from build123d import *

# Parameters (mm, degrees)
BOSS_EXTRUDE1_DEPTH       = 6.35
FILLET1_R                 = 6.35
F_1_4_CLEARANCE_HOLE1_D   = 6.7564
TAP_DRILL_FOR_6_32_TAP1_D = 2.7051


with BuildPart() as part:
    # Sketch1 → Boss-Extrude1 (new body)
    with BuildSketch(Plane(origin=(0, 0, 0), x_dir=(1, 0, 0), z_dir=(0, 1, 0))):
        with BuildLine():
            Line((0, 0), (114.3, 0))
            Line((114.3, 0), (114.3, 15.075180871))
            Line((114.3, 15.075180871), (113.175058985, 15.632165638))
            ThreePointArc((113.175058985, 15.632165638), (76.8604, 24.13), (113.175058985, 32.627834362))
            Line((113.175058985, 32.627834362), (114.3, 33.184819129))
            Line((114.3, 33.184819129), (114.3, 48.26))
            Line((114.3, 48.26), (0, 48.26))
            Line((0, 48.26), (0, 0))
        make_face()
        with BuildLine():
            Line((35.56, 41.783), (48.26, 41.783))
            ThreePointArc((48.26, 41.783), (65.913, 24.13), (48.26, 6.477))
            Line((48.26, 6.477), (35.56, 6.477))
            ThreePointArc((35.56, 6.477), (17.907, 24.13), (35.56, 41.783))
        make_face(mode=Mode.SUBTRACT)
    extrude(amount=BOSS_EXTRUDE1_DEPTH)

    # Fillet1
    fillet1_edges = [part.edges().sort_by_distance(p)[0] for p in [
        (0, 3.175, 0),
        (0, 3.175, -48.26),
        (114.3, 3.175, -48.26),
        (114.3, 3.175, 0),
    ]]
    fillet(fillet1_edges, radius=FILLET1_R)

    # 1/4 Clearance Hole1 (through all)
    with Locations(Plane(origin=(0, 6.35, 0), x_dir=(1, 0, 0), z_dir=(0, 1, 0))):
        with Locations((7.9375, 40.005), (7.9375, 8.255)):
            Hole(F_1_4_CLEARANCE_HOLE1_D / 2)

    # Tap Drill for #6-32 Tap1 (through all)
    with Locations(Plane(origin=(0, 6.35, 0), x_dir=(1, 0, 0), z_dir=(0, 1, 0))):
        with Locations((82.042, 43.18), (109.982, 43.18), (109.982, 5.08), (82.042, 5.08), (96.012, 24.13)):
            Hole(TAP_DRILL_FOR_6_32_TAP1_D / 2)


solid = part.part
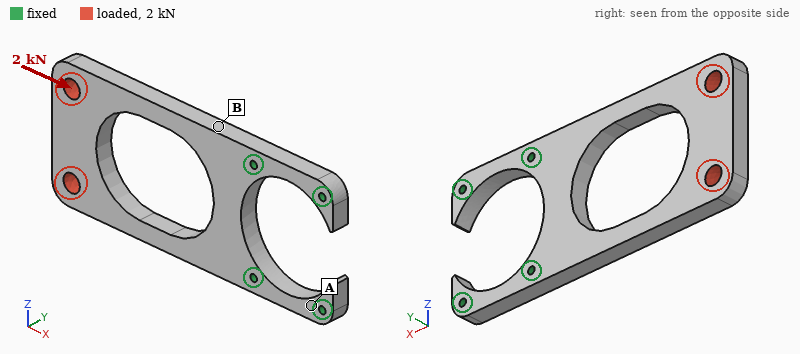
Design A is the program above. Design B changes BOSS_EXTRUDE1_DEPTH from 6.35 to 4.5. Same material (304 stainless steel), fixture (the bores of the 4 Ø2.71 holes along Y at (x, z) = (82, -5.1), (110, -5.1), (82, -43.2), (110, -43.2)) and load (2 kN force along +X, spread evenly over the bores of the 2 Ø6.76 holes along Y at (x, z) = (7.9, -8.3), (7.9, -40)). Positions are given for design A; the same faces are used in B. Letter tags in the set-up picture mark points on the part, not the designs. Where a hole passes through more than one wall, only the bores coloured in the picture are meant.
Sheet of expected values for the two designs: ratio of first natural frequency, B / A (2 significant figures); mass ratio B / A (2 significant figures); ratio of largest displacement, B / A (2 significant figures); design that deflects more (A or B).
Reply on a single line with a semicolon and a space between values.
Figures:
0.72; 0.71; 1.4; B
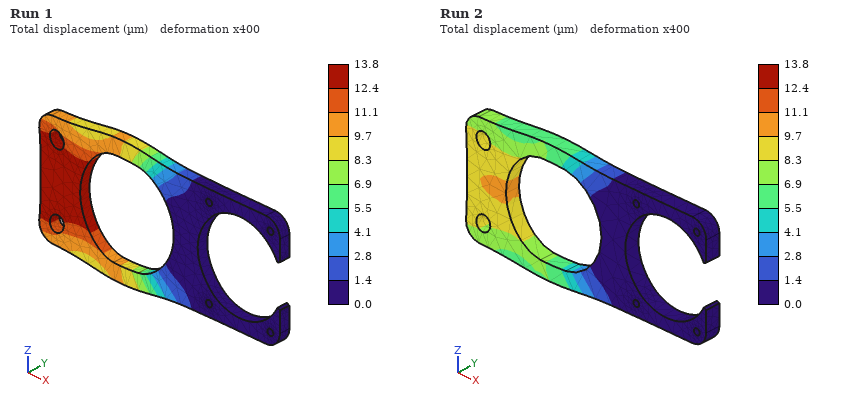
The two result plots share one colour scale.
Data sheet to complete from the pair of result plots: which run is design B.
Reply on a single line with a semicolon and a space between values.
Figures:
Run 1
